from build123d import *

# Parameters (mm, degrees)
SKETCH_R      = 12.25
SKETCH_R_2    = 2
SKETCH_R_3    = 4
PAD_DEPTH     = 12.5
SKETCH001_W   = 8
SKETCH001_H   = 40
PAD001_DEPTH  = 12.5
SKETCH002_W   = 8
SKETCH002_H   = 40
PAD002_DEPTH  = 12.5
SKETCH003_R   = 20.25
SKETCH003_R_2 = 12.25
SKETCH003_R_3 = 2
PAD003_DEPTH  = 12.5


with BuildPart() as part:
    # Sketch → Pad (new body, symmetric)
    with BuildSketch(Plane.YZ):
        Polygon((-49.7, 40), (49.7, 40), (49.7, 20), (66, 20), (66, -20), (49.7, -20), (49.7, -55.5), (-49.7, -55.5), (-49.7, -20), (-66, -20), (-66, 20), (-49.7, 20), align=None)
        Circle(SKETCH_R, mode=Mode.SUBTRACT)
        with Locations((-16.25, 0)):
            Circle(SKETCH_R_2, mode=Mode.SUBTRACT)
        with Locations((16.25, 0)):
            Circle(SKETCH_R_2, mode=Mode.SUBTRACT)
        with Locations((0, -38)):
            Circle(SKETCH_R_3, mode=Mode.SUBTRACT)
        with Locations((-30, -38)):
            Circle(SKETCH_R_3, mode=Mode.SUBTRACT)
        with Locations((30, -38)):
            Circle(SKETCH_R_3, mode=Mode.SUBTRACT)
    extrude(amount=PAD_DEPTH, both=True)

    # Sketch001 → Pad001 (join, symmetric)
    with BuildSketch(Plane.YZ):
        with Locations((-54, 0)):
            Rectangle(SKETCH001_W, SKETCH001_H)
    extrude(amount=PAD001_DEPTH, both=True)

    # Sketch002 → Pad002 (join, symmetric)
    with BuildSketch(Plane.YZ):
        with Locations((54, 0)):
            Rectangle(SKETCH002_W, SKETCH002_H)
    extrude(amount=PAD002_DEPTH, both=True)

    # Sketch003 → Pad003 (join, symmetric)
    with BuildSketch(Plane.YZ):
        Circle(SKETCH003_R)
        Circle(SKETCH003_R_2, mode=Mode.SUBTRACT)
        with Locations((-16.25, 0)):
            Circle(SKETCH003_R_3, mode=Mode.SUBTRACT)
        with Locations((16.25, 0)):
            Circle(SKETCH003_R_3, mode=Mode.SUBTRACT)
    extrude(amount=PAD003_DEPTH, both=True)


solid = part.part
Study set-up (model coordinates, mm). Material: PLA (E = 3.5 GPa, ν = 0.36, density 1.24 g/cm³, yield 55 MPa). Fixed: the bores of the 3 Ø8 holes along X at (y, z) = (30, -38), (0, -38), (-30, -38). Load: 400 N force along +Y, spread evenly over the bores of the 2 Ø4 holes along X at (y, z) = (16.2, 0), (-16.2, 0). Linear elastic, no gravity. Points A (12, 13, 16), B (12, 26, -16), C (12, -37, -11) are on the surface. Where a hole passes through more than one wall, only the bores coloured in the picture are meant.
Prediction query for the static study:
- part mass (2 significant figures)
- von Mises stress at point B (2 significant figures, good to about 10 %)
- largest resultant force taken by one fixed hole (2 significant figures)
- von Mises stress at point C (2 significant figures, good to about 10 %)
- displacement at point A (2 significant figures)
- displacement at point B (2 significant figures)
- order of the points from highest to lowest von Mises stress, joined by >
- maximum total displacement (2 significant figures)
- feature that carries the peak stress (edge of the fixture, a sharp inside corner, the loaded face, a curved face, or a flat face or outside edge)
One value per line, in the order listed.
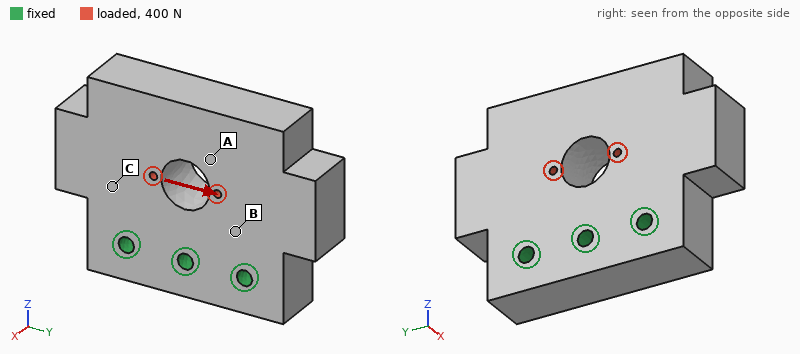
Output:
310 g
0.41 MPa
250 N
0.26 MPa
11 µm
4.5 µm
B > C > A
15 µm
the loaded face
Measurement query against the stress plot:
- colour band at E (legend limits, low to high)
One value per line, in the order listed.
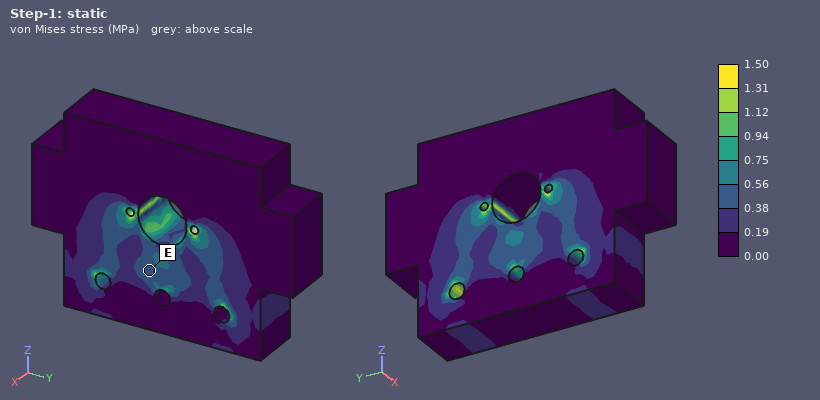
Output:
0.38 to 0.56 MPa
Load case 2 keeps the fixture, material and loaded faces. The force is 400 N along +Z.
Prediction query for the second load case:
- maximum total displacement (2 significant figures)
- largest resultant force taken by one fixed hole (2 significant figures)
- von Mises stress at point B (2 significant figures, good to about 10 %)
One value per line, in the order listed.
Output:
4.0 µm
150 N
0.27 MPa
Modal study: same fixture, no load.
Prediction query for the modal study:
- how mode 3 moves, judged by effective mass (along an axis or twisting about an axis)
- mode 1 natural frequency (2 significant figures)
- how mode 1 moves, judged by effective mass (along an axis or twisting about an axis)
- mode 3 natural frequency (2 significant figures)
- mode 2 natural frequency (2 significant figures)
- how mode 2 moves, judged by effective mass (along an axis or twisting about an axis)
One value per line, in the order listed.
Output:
along Y
940 Hz
along X
1700 Hz
1400 Hz
twisting about Z
